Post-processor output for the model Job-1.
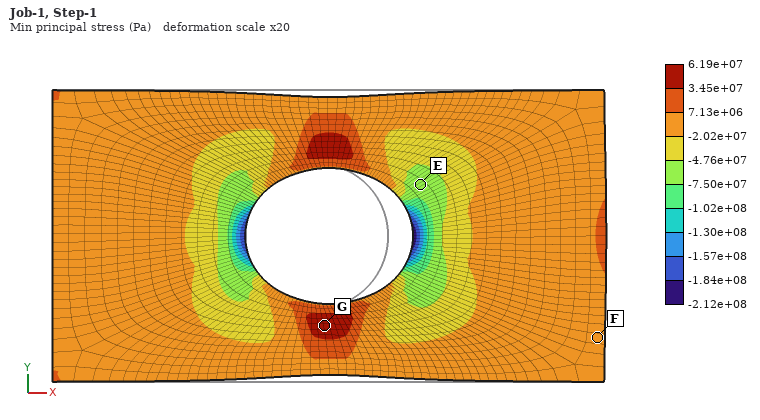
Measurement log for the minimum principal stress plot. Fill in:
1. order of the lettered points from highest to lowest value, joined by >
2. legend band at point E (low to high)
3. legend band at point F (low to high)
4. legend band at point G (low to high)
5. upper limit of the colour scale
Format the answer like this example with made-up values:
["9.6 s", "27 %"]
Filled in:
["G > F > E", "-7.50e+07 to -4.76e+07 Pa", "-2.02e+07 to 7.13e+06 Pa", "3.45e+07 to 6.19e+07 Pa", "6.19e+07 Pa"]
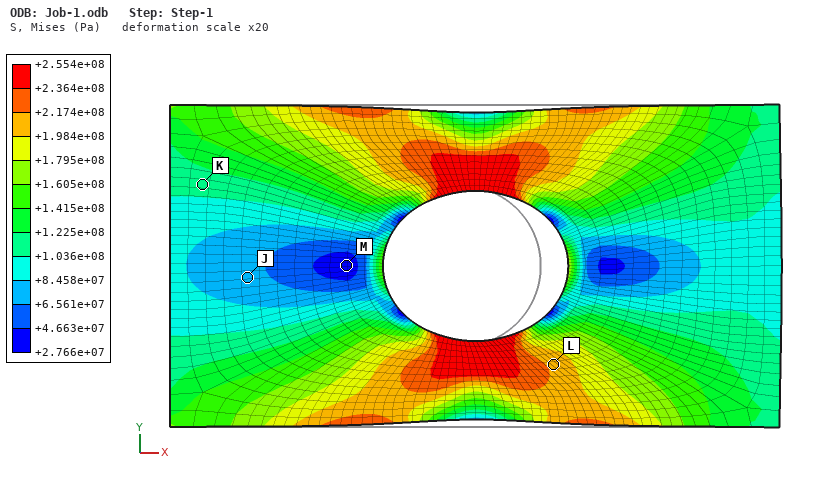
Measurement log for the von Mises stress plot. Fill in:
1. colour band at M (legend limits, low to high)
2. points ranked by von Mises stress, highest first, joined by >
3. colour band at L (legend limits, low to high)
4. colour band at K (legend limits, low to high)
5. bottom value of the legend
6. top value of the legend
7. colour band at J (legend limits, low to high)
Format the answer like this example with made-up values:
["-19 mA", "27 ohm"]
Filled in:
["+2.766e+07 to +4.663e+07 Pa", "L > K > J > M", "+1.984e+08 to +2.174e+08 Pa", "+1.036e+08 to +1.225e+08 Pa", "+2.766e+07 Pa", "+2.554e+08 Pa", "+6.561e+07 to +8.458e+07 Pa"]
